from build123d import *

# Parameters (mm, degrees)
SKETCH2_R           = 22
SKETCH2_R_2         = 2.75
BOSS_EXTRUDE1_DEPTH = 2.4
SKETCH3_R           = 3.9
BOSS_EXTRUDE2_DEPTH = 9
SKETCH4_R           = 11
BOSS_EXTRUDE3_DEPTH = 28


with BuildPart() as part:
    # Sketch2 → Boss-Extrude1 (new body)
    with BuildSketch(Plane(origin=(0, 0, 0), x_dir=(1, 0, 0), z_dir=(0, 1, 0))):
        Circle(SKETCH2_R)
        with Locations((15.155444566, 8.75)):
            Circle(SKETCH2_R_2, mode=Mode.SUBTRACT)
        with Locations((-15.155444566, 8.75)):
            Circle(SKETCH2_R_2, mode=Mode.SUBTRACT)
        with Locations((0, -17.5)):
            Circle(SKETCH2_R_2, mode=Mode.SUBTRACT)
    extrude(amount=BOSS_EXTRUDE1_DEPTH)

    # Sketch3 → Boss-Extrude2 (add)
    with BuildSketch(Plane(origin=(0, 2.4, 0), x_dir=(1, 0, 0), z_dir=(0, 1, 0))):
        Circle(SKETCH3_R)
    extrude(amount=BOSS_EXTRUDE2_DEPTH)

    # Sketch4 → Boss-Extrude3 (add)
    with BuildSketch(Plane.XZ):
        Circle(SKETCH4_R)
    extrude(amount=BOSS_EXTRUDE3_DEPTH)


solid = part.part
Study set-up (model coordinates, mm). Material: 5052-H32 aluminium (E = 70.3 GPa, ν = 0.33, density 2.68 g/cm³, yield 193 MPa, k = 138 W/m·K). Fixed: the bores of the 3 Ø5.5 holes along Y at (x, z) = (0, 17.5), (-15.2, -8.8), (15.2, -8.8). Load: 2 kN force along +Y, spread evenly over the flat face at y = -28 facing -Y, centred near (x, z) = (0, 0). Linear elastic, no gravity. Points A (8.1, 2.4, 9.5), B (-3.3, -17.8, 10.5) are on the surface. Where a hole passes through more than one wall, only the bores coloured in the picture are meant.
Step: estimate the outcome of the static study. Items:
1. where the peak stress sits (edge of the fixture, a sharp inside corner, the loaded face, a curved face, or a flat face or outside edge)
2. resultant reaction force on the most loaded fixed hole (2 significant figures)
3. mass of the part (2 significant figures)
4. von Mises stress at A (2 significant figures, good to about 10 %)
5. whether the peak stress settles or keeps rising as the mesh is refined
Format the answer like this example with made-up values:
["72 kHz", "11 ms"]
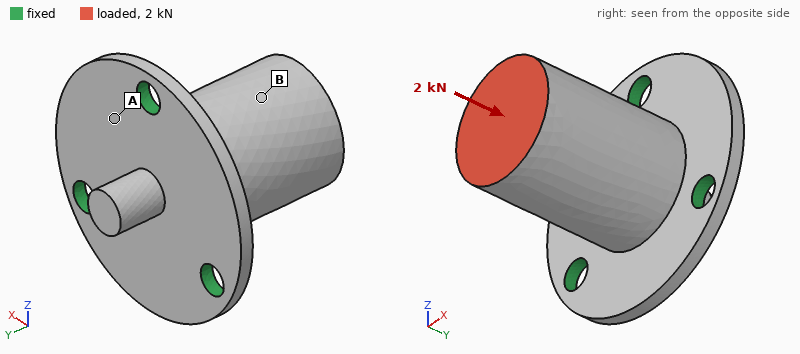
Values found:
["edge of the fixture", "720 N", "39 g", "26 MPa", "keeps rising"]
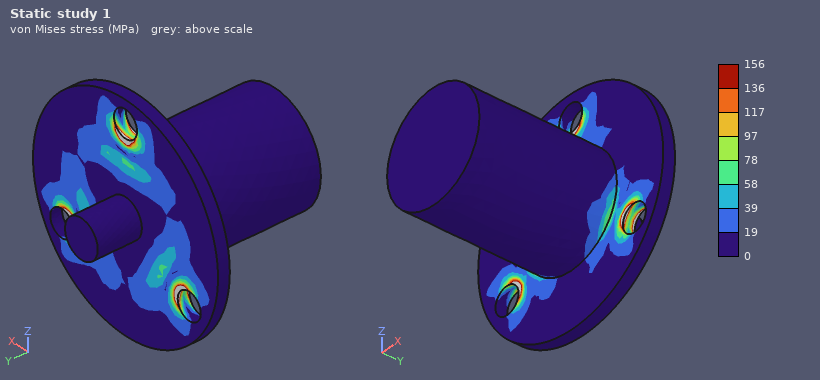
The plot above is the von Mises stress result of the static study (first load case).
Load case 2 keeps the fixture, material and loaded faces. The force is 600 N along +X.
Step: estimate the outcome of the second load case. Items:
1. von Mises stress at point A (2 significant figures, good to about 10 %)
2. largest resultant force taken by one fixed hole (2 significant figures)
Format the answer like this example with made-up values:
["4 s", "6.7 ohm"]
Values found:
["15 MPa", "760 N"]
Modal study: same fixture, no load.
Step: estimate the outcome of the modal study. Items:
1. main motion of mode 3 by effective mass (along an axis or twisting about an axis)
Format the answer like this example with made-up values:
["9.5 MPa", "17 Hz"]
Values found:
["along Y"]
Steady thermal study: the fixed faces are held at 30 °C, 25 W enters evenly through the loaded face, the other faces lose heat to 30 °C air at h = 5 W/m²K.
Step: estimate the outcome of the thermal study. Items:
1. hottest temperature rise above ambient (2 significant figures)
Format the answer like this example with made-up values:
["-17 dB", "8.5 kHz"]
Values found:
["24 K"]
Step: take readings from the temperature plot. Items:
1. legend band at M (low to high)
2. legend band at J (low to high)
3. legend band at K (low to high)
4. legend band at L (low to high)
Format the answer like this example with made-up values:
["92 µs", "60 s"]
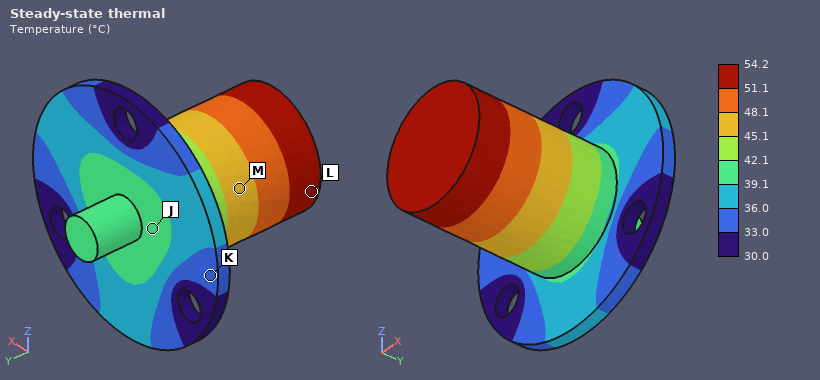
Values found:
["45.1 to 48.1 °C", "39.1 to 42.1 °C", "33.0 to 36.0 °C", "51.1 to 54.2 °C"]
